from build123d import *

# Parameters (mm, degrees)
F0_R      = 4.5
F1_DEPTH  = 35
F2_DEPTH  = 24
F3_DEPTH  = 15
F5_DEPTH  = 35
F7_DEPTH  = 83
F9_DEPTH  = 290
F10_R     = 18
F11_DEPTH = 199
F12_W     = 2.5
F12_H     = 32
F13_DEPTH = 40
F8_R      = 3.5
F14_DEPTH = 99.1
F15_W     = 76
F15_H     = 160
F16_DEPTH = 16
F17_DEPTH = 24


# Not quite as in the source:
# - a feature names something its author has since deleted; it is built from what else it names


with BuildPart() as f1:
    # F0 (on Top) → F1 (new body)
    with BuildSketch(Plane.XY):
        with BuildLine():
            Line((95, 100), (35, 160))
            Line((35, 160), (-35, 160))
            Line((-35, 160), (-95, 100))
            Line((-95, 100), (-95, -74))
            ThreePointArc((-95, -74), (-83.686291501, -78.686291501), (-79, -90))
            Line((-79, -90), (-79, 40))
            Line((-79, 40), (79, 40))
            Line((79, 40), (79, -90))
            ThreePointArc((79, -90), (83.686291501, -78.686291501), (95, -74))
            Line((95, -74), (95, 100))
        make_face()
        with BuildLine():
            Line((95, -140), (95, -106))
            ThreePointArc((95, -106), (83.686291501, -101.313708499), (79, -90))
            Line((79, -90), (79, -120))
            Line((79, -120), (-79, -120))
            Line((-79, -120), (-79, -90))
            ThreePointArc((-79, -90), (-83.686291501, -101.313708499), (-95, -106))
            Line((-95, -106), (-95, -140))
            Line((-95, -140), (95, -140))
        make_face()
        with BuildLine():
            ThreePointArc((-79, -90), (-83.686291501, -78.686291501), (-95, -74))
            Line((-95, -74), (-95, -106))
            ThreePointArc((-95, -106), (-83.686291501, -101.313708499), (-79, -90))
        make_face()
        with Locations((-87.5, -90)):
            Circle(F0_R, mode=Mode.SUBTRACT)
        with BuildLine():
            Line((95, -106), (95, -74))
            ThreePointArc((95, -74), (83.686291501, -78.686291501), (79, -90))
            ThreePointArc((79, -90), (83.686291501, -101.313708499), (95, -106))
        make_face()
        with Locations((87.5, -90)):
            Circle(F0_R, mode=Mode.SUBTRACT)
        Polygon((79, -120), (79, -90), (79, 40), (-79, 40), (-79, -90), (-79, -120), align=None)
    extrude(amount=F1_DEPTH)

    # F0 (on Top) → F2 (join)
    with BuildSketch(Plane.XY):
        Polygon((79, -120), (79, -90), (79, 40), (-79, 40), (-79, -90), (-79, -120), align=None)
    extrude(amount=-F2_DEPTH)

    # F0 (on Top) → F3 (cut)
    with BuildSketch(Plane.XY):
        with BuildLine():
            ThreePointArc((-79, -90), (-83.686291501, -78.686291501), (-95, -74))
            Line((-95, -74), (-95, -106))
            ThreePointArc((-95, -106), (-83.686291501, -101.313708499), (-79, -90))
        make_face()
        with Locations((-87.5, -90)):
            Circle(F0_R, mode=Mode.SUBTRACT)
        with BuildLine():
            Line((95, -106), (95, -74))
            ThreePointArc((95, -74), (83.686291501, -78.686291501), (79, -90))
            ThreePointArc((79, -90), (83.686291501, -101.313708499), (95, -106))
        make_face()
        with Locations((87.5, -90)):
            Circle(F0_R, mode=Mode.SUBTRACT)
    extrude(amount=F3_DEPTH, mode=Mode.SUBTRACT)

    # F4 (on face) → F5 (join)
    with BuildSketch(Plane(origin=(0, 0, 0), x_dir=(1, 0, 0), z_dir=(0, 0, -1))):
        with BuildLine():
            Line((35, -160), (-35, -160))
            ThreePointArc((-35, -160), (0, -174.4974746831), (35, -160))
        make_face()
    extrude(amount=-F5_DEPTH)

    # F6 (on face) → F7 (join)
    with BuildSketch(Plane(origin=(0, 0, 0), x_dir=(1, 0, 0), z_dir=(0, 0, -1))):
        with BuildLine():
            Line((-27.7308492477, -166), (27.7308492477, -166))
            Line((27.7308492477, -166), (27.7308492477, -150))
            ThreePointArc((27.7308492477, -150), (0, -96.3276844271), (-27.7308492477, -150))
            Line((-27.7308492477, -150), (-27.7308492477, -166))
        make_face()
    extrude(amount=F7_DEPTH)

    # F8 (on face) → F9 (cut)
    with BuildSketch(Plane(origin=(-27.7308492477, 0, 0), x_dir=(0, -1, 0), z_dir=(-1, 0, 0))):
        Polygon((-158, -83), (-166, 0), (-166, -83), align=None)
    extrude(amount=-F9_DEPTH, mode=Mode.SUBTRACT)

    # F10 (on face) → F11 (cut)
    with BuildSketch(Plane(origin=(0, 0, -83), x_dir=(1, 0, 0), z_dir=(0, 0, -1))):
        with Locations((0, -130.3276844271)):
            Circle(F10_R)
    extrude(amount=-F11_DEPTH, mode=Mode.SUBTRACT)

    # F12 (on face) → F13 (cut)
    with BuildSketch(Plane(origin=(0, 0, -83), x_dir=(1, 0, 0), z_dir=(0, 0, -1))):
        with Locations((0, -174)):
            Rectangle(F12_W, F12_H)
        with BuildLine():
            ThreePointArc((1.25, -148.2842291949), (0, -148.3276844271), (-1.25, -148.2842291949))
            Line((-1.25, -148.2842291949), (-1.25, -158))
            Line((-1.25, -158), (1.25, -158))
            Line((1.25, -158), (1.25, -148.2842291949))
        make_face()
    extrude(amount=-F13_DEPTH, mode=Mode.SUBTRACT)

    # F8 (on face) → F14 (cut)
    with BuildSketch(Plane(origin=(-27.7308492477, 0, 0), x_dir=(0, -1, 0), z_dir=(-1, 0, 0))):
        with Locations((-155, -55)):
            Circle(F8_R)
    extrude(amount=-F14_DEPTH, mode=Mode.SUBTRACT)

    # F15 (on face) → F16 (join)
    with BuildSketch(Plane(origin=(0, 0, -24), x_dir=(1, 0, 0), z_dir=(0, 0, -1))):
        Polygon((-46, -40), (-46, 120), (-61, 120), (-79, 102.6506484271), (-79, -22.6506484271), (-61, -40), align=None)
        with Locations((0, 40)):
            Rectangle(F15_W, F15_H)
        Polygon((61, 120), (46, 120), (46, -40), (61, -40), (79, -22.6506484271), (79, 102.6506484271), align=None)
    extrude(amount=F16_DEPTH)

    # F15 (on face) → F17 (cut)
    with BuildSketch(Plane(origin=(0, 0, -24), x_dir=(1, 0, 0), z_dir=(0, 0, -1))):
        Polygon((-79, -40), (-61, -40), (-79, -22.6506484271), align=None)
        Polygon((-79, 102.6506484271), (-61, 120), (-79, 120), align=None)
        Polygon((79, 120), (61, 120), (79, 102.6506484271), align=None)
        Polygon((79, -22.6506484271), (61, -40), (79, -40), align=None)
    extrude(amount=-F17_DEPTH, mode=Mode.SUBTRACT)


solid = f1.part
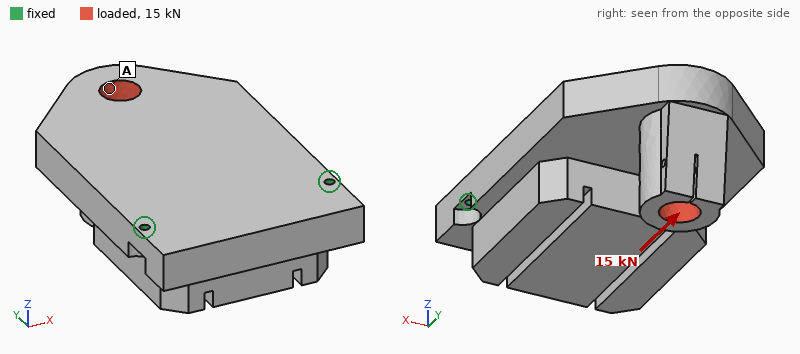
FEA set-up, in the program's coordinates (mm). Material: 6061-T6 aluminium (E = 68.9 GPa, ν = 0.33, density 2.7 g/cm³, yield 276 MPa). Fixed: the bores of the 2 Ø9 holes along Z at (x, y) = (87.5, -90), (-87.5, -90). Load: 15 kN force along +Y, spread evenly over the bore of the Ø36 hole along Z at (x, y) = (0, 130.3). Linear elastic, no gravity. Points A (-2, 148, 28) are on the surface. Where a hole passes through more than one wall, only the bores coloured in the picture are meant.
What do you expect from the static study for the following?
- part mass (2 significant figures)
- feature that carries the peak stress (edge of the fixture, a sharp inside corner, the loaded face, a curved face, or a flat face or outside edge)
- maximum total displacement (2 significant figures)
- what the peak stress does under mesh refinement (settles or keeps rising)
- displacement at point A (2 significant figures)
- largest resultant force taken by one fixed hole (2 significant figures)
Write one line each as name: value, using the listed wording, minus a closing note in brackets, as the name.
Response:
part mass: 8.1 kg
feature that carries the peak stress: edge of the fixture
maximum total displacement: 0.83 mm
what the peak stress does under mesh refinement: keeps rising
displacement at point A: 0.66 mm
largest resultant force taken by one fixed hole: 7.5 kN
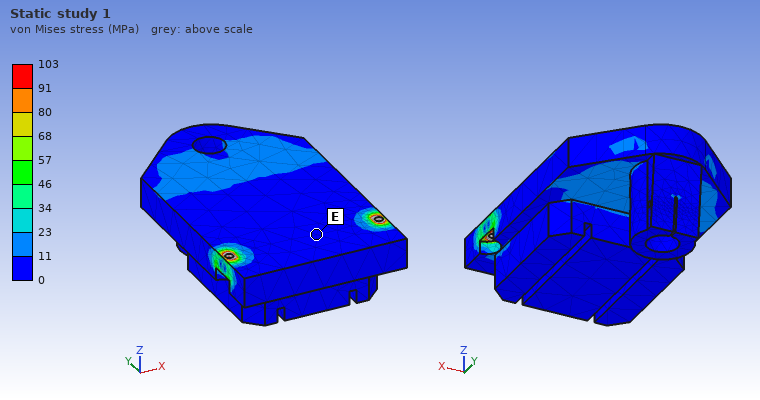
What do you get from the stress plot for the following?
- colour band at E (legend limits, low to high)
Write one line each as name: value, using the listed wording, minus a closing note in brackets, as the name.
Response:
colour band at E: 0 to 11 MPa
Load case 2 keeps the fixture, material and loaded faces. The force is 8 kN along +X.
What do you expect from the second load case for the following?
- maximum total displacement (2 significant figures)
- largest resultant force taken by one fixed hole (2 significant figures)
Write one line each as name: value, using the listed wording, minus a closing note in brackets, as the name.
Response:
maximum total displacement: 0.11 mm
largest resultant force taken by one fixed hole: 11 kN
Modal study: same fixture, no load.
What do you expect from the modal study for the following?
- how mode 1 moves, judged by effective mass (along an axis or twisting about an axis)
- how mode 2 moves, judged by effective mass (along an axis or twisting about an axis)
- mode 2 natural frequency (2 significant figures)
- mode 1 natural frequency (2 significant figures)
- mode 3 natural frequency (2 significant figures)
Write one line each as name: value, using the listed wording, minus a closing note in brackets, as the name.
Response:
how mode 1 moves, judged by effective mass: along Z
how mode 2 moves, judged by effective mass: along X
mode 2 natural frequency: 1400 Hz
mode 1 natural frequency: 250 Hz
mode 3 natural frequency: 1600 Hz
